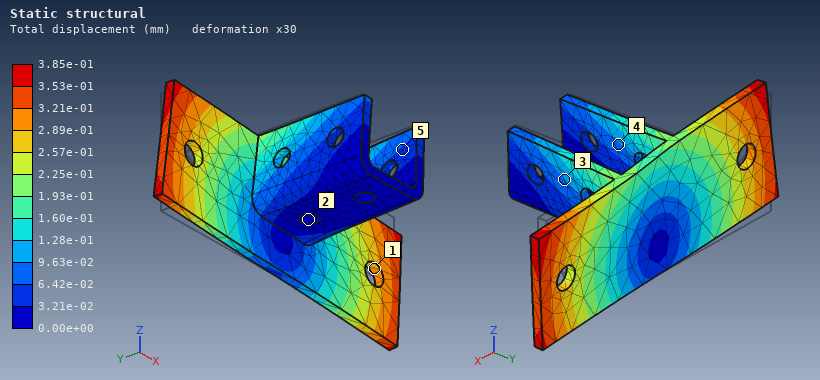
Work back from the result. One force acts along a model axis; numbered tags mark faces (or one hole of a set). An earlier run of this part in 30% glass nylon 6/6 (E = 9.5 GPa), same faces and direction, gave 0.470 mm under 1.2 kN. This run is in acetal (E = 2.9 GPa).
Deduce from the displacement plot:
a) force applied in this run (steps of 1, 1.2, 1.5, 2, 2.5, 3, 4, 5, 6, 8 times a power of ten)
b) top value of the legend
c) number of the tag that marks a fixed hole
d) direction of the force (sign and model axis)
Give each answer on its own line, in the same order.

300 N
3.85e-01 mm
2
+X
